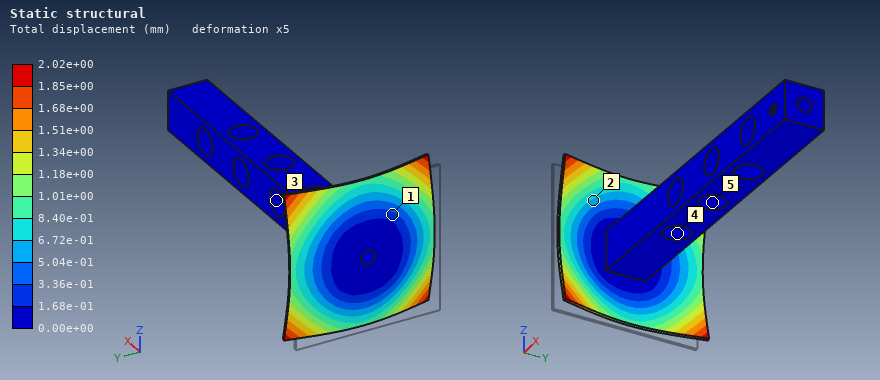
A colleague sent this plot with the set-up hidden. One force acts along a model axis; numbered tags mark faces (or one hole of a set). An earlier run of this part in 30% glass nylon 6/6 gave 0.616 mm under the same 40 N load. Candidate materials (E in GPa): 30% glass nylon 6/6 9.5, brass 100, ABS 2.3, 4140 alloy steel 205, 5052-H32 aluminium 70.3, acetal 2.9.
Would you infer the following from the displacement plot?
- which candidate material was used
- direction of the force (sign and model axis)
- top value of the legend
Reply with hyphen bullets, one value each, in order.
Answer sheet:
- acetal
- +X
- 2.02e+00 mm
